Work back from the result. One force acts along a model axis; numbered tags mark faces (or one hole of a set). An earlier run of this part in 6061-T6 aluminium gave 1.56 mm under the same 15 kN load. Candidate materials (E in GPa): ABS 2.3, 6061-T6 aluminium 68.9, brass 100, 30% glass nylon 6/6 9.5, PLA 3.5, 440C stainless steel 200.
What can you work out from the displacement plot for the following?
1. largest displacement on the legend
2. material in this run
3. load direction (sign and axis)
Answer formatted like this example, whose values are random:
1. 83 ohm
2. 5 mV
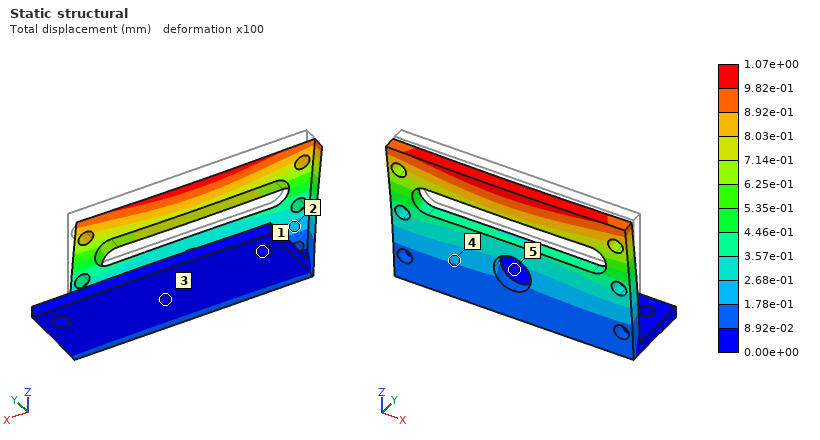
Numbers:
1. 1.07e+00 mm
2. brass
3. -Y
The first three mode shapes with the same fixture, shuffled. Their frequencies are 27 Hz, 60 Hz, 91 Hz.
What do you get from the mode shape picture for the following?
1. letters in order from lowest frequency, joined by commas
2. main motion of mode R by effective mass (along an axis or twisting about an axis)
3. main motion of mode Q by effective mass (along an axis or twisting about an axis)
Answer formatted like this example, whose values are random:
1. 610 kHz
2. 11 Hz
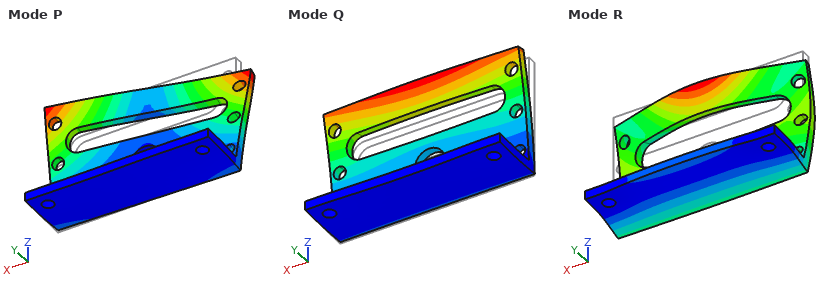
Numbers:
1. Q, P, R
2. along Z
3. along Y
